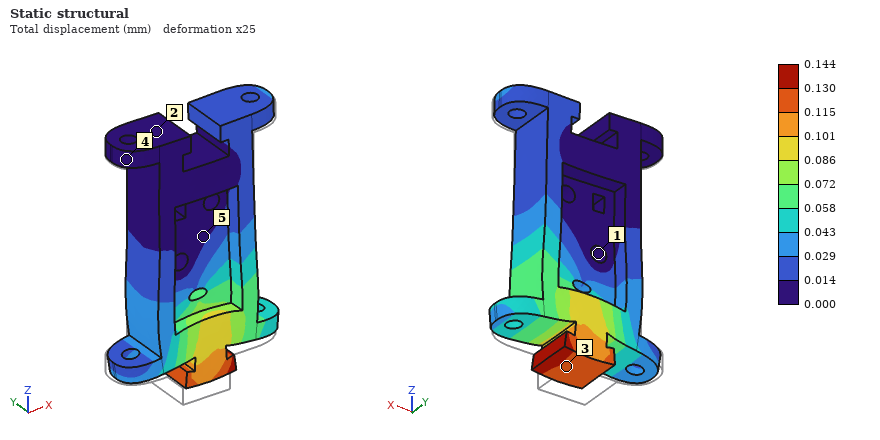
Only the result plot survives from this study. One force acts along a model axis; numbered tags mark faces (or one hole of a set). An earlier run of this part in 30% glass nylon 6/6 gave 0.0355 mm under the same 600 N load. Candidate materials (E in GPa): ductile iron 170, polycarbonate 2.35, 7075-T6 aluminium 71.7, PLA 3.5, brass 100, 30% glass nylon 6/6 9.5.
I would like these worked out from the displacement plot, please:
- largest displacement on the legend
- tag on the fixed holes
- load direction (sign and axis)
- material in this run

0.144 mm
1
+Z
polycarbonate
